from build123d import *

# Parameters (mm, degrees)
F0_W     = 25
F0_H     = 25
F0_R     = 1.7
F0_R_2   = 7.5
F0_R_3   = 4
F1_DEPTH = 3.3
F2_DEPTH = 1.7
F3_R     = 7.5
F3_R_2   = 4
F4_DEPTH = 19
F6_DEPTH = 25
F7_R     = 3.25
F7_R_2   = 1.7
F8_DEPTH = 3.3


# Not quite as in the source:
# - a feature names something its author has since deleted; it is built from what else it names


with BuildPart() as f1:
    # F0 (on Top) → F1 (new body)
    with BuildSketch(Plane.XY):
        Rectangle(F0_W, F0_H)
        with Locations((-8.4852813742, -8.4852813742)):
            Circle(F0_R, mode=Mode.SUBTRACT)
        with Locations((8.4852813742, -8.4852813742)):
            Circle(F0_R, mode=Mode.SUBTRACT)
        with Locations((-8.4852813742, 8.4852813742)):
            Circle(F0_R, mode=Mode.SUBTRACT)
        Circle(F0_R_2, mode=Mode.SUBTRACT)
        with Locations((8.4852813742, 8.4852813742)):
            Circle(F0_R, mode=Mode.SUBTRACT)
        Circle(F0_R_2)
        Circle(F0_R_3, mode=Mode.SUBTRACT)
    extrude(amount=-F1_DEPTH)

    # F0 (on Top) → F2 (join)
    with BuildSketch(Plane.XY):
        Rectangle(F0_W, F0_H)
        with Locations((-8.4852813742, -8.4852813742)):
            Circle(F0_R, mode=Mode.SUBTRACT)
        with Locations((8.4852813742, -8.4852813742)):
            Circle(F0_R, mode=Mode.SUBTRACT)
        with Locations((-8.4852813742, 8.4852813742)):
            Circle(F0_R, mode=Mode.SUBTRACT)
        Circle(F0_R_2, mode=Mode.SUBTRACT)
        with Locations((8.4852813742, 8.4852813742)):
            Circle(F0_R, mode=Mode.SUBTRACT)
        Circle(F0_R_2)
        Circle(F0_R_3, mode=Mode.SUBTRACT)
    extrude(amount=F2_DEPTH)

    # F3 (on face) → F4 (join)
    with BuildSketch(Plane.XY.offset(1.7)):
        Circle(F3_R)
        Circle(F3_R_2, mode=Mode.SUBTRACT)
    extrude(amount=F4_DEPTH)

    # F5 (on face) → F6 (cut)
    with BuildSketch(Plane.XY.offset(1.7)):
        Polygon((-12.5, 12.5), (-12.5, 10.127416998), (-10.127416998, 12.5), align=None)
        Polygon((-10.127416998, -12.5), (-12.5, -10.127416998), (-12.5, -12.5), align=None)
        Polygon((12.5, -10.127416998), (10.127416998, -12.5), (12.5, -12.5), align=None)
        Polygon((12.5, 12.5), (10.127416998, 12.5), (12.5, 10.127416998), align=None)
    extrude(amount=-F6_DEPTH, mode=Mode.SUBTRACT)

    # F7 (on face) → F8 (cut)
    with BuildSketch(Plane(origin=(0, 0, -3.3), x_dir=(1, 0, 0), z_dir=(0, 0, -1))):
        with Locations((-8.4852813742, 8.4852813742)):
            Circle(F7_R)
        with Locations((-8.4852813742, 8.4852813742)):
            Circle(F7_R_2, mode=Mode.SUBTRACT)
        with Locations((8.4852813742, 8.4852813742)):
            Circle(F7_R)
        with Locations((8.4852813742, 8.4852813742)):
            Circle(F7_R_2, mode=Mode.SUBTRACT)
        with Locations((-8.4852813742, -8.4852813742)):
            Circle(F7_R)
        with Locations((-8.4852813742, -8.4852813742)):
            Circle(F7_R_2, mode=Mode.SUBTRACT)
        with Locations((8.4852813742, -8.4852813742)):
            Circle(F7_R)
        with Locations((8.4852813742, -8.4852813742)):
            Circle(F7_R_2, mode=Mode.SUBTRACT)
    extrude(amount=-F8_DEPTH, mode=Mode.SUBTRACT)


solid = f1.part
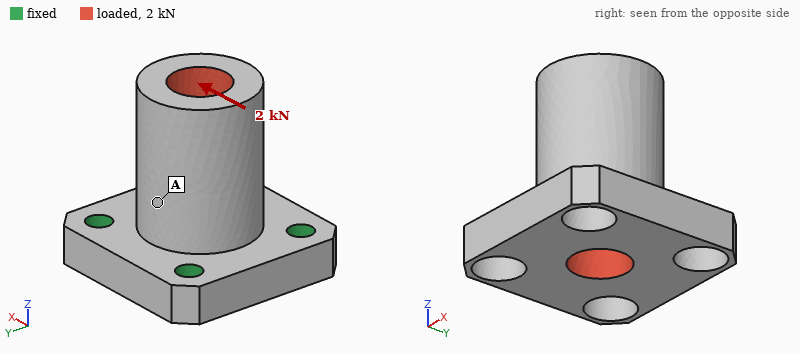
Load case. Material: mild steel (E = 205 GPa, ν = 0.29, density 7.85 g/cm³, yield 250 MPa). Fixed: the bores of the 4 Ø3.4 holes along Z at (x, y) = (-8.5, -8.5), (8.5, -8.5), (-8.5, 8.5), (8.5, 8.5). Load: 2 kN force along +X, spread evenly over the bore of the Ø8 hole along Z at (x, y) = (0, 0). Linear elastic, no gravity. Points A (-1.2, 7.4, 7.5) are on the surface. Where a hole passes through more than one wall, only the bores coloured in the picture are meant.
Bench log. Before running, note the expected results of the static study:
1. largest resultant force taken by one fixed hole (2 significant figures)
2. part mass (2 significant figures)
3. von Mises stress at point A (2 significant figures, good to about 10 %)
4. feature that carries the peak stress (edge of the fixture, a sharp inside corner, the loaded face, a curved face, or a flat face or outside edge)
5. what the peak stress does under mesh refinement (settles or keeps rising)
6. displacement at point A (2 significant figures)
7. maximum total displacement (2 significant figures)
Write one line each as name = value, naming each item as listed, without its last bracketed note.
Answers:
largest resultant force taken by one fixed hole = 690 N
part mass = 37 g
von Mises stress at point A = 19 MPa
feature that carries the peak stress = edge of the fixture
what the peak stress does under mesh refinement = keeps rising
displacement at point A = 5.3 µm
maximum total displacement = 15 µm
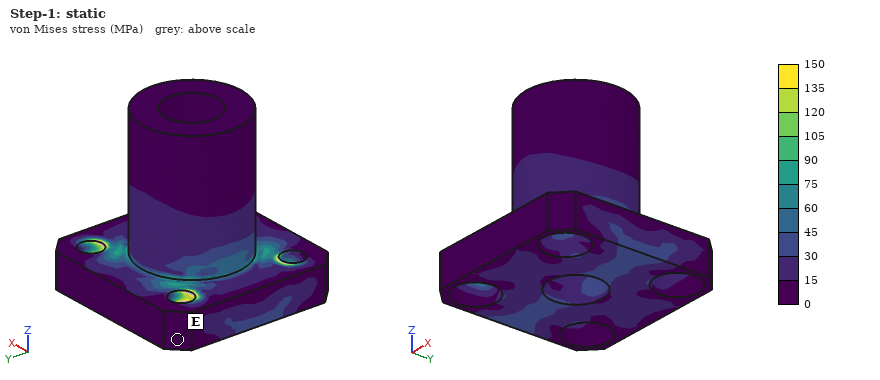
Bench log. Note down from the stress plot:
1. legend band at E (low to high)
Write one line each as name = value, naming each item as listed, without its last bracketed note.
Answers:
legend band at E = 0 to 15 MPa
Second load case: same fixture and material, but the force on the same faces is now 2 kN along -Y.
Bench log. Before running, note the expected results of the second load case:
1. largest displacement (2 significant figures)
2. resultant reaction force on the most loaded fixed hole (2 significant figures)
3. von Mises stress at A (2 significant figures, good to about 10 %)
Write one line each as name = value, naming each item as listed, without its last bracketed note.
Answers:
largest displacement = 15 µm
resultant reaction force on the most loaded fixed hole = 690 N
von Mises stress at A = 21 MPa
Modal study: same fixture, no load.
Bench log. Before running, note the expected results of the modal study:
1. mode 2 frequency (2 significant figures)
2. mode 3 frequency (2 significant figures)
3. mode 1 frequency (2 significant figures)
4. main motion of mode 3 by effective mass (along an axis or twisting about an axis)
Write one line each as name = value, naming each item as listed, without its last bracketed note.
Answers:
mode 2 frequency = 14 kHz
mode 3 frequency = 25 kHz
mode 1 frequency = 14 kHz
main motion of mode 3 by effective mass = along Z
